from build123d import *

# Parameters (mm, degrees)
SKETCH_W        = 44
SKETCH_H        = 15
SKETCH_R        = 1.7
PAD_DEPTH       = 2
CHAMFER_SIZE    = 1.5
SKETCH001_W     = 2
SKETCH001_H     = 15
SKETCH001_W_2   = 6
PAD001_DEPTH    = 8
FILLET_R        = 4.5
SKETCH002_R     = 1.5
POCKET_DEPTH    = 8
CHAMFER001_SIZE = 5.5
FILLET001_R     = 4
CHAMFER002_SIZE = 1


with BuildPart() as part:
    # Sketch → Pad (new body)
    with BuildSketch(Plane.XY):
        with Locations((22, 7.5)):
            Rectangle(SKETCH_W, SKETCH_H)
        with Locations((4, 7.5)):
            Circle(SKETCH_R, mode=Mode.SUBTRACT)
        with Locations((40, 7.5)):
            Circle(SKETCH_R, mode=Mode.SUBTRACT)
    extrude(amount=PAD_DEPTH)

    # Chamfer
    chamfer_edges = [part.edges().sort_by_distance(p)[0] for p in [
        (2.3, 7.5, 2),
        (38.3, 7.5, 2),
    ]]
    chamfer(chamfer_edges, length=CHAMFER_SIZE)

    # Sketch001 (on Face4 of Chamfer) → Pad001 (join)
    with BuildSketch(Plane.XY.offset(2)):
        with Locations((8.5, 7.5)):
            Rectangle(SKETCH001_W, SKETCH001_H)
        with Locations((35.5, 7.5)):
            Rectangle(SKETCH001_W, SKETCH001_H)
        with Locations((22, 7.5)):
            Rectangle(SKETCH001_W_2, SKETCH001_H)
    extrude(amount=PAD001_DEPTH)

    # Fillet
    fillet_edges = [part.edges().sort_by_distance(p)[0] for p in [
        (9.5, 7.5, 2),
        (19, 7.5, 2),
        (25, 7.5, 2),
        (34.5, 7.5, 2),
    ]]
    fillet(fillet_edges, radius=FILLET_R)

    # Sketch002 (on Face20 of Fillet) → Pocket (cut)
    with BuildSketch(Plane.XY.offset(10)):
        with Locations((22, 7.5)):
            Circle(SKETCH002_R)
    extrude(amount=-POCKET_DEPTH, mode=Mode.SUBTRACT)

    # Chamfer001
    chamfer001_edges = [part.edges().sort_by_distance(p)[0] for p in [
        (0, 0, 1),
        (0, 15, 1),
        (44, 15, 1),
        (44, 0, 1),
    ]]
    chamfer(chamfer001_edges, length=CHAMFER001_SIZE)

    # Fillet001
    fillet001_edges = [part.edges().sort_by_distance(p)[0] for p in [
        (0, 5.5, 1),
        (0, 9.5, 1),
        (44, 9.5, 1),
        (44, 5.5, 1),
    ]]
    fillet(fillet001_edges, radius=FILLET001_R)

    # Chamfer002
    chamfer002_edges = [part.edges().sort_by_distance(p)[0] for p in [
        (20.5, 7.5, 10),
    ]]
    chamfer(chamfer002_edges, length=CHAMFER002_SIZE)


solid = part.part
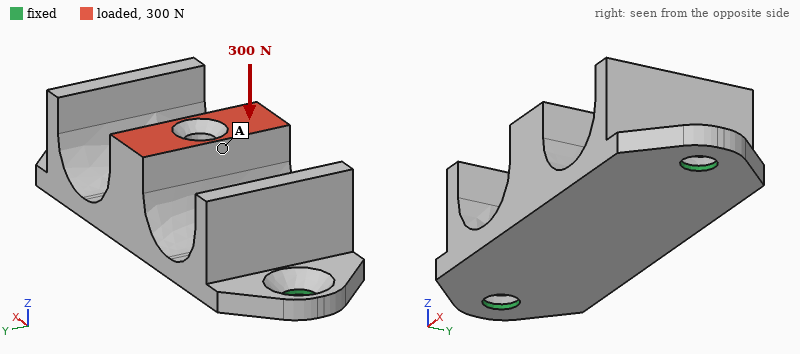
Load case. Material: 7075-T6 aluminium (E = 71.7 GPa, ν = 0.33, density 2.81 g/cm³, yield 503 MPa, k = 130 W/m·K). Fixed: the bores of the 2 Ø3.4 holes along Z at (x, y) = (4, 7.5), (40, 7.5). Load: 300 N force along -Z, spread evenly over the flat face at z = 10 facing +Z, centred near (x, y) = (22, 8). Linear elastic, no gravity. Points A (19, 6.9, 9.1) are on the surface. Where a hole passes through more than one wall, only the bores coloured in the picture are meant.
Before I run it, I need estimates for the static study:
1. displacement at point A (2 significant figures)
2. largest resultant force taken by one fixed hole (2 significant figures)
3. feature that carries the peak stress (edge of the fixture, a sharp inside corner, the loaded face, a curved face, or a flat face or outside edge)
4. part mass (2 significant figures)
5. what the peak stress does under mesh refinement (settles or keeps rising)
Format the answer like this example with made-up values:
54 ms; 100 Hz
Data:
54 µm; 400 N; edge of the fixture; 7.1 g; keeps rising
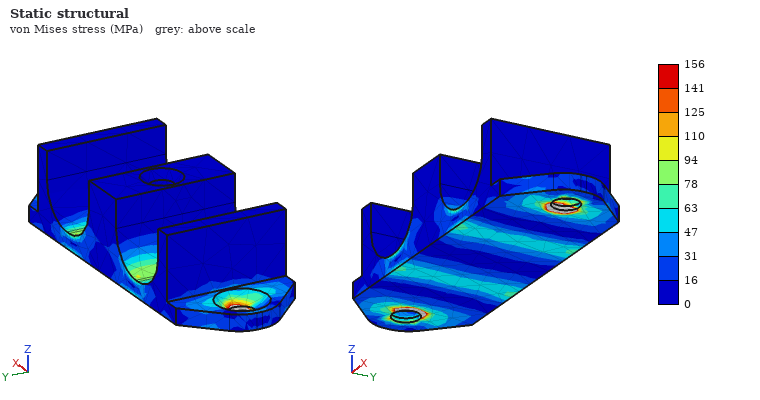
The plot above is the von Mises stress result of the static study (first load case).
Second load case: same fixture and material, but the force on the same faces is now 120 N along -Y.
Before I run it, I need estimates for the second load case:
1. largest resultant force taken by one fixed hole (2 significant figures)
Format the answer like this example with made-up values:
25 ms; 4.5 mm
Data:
60 N
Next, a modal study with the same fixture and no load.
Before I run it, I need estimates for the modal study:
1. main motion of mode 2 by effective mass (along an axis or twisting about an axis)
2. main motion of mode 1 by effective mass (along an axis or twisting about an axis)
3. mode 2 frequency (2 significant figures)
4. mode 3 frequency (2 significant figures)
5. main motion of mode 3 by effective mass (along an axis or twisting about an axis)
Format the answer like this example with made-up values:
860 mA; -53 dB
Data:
along Z; along Y; 5600 Hz; 12 kHz; twisting about Y
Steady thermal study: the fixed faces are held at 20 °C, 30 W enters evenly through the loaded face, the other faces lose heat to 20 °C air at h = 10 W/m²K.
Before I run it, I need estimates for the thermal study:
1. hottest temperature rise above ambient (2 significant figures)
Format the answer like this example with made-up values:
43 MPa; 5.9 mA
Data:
82 K
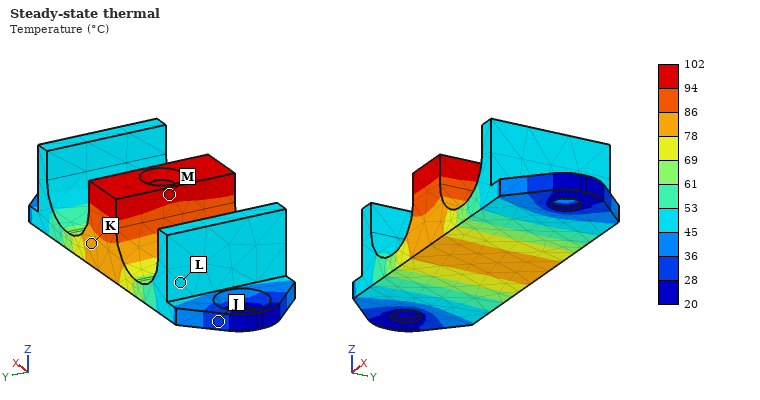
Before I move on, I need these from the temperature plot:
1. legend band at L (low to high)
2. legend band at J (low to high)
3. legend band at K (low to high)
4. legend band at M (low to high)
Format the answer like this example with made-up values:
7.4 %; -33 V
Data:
45 to 53 °C; 28 to 36 °C; 78 to 86 °C; 94 to 102 °C
